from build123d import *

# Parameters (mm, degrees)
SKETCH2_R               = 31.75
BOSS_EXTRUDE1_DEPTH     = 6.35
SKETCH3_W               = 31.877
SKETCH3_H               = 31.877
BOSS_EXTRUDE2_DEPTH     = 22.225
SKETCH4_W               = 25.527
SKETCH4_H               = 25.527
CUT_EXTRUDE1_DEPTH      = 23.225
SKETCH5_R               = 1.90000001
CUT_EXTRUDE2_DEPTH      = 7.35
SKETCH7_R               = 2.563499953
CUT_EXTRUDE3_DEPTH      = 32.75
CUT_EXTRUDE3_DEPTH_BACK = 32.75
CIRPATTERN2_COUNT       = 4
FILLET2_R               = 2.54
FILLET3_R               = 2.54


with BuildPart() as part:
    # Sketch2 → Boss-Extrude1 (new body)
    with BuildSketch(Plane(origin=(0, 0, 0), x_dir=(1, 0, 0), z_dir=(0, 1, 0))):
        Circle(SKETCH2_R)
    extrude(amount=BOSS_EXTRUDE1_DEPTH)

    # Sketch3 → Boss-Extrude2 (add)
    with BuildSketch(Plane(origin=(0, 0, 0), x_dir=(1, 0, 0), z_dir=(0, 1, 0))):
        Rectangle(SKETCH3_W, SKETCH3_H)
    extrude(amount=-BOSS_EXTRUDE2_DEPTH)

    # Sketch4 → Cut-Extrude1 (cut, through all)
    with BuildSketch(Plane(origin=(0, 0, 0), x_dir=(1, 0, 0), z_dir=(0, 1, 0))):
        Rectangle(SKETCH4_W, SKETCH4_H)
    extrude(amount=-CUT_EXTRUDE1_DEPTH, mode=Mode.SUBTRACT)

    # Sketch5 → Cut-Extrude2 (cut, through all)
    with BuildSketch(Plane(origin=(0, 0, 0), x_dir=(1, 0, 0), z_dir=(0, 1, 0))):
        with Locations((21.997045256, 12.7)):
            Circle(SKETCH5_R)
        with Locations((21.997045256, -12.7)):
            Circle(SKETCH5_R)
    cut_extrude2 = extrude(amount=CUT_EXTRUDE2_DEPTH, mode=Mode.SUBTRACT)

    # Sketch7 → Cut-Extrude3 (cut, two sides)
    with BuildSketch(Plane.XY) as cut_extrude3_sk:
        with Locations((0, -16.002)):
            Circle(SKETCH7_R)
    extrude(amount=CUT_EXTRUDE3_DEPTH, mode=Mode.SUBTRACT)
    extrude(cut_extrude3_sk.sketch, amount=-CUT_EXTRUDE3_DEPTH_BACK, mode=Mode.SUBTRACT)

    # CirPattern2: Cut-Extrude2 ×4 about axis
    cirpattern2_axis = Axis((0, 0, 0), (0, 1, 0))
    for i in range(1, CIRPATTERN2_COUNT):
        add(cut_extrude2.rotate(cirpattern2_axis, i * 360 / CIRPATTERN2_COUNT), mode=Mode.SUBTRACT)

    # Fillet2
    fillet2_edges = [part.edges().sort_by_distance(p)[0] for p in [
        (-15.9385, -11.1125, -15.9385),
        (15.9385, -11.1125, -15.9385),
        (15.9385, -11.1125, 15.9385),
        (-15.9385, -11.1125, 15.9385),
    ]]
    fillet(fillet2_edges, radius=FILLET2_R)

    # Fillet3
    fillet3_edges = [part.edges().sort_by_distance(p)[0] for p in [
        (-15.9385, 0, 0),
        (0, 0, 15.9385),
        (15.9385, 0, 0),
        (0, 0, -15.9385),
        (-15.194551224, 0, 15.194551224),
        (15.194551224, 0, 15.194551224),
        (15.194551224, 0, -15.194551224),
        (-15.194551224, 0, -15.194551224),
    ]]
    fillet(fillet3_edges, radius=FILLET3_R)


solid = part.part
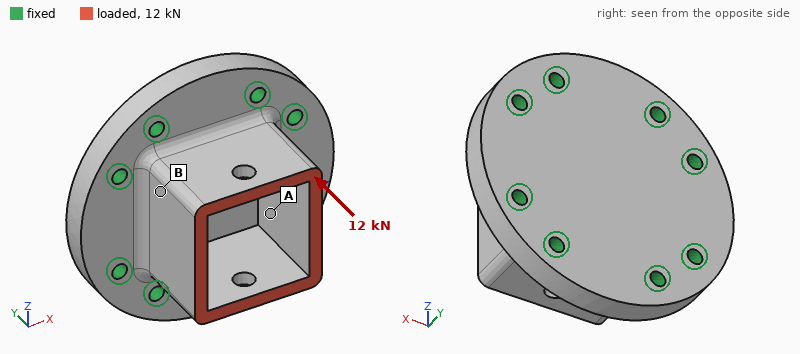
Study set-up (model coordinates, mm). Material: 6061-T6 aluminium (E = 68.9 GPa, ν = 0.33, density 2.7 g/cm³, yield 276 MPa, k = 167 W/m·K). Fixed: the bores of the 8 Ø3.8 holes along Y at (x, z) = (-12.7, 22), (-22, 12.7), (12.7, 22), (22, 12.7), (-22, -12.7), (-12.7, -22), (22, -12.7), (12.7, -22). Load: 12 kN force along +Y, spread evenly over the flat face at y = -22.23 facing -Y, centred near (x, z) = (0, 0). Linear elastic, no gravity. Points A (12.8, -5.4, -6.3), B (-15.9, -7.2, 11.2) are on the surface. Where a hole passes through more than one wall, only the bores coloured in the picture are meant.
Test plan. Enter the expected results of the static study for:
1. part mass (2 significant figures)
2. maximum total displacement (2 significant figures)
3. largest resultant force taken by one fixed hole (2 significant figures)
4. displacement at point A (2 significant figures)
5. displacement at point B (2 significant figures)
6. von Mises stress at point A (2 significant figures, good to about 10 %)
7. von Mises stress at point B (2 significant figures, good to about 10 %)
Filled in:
74 g
25 µm
1.6 kN
14 µm
14 µm
21 MPa
43 MPa
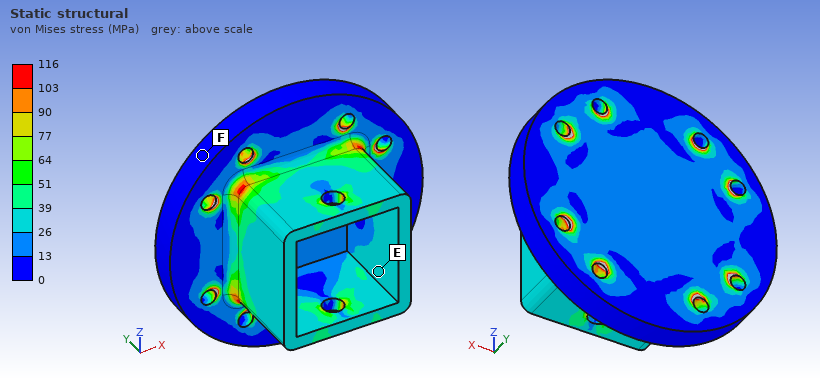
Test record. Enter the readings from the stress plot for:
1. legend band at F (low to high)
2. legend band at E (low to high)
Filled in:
0 to 13 MPa
26 to 39 MPa
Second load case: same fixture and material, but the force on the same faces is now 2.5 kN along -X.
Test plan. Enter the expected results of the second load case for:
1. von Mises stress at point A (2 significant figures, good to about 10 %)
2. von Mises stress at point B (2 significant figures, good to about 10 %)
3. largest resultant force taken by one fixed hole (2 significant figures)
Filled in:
20 MPa
27 MPa
730 N
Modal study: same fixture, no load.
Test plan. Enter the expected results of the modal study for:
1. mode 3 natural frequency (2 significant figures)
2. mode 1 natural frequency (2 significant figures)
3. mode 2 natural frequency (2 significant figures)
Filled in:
16 kHz
13 kHz
15 kHz
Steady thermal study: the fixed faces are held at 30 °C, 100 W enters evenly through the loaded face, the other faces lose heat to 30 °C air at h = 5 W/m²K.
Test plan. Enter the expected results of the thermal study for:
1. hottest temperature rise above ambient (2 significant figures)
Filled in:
48 K
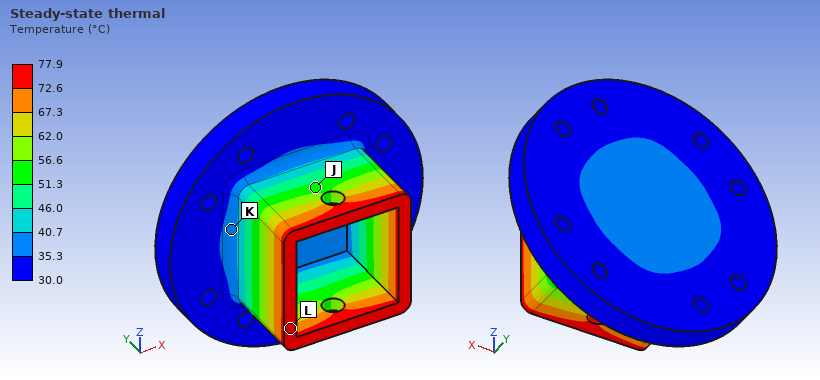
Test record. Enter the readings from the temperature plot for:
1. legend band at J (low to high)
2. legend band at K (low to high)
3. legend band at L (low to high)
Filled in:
51.3 to 56.6 °C
35.3 to 40.7 °C
72.6 to 77.9 °C
